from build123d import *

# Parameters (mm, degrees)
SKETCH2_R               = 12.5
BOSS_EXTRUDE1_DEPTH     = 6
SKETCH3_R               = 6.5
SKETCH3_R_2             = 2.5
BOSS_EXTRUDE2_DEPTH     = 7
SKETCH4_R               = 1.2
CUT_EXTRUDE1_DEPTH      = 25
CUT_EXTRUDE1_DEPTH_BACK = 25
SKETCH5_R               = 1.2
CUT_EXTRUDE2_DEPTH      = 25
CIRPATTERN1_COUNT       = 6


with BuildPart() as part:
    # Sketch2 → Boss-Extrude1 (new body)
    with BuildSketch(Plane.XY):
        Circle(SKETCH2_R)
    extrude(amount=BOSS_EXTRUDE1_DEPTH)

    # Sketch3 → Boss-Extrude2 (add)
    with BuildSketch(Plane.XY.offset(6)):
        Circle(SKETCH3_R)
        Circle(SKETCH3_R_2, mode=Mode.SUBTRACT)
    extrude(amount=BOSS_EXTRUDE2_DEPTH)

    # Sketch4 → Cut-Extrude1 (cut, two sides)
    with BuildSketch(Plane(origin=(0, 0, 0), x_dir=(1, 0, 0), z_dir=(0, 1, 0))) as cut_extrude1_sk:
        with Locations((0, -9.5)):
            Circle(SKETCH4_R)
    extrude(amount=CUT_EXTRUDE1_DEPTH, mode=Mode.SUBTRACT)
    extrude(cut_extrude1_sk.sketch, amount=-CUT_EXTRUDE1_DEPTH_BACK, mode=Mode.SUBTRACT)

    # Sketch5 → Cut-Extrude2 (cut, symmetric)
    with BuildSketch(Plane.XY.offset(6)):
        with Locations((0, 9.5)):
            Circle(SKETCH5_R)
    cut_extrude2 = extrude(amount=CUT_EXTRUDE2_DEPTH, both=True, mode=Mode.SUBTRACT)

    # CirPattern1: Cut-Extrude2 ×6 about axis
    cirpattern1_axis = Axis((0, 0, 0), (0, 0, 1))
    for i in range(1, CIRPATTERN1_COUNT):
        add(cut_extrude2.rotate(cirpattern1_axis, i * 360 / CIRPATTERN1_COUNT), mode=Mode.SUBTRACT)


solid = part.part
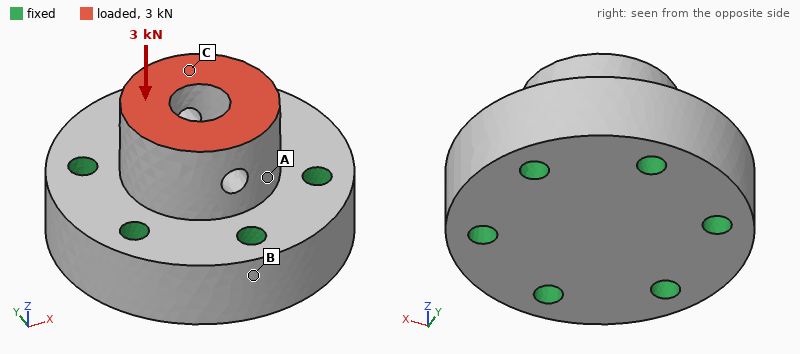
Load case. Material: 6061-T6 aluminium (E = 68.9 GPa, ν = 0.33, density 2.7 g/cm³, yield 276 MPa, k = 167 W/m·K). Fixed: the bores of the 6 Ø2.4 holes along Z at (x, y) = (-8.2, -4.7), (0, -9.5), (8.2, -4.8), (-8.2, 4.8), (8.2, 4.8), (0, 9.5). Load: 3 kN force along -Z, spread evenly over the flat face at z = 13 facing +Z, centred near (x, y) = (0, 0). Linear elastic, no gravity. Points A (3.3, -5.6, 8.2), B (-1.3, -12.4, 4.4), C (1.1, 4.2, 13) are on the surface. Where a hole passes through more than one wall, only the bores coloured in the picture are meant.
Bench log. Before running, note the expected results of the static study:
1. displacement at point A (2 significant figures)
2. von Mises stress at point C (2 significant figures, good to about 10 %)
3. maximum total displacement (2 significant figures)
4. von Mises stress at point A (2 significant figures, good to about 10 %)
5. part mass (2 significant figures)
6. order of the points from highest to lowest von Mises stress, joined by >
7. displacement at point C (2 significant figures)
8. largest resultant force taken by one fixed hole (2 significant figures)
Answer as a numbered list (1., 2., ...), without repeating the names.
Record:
1. 3.8 µm
2. 24 MPa
3. 6.8 µm
4. 35 MPa
5. 9.6 g
6. A > C > B
7. 6.1 µm
8. 540 N
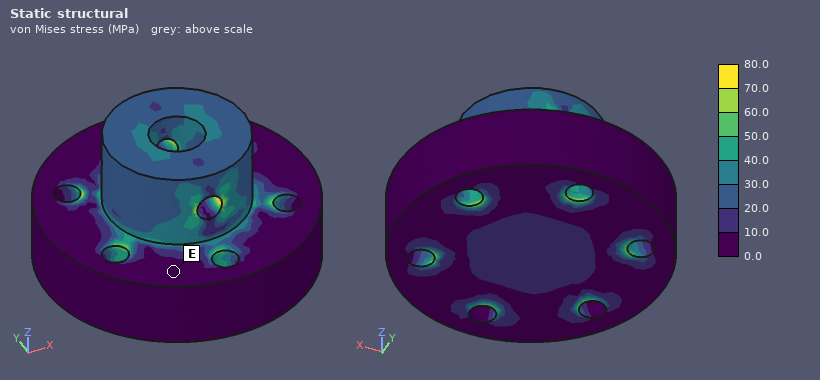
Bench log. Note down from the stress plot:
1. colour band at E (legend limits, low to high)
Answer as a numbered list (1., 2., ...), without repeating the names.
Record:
1. 0.0 to 10.0 MPa
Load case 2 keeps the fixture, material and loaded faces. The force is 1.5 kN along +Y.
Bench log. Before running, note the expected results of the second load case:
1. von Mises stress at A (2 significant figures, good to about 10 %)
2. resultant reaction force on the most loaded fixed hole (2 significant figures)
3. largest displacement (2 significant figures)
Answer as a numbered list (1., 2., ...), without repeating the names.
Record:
1. 43 MPa
2. 660 N
3. 15 µm
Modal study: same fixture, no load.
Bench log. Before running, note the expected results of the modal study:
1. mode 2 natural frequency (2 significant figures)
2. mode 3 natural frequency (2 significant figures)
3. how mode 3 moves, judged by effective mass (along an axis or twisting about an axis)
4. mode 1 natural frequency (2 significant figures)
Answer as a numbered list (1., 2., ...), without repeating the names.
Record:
1. 61 kHz
2. 76 kHz
3. along Z
4. 59 kHz
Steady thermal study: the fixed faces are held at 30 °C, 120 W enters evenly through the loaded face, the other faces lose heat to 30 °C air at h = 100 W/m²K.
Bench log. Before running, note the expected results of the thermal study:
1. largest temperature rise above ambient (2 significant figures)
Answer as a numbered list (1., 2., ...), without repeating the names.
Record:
1. 69 K
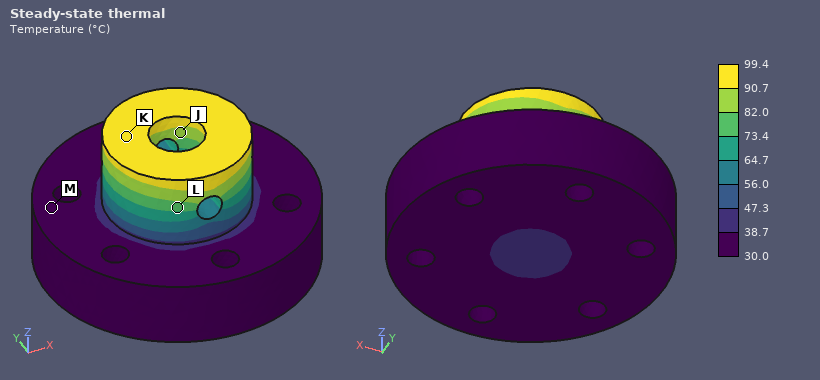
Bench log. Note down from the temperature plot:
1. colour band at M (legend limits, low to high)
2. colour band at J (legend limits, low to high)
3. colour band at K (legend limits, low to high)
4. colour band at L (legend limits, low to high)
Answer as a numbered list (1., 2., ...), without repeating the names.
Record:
1. 30.0 to 38.7 °C
2. 82.0 to 90.7 °C
3. 90.7 to 99.4 °C
4. 73.4 to 82.0 °C
